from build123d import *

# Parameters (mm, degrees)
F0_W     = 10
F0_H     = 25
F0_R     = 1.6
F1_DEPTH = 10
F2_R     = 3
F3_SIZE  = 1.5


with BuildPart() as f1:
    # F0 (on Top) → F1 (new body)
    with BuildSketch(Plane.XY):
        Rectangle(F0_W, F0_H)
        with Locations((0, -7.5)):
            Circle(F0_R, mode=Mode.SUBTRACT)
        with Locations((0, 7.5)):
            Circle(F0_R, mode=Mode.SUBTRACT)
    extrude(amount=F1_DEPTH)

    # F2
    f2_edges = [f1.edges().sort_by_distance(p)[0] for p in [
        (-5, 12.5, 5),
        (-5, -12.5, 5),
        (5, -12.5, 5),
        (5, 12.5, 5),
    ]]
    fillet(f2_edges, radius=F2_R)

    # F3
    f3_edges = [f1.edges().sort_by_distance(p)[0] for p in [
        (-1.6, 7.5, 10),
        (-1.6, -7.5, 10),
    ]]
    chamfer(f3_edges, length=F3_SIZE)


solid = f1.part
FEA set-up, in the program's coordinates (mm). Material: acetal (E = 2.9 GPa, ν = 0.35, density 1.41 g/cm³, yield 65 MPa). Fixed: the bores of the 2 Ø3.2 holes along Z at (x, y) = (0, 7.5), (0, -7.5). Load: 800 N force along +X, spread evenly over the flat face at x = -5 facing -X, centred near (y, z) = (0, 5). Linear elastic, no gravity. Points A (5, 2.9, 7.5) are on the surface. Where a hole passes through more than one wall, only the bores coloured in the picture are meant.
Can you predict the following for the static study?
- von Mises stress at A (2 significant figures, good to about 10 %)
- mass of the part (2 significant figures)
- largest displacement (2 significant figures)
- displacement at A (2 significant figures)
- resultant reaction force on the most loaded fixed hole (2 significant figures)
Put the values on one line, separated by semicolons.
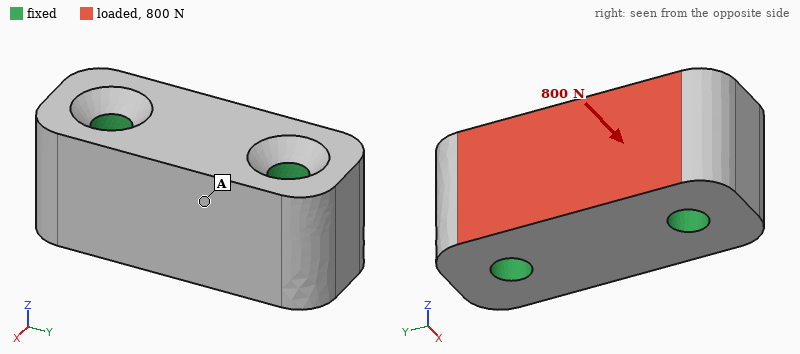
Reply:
3.1 MPa; 3.1 g; 24 µm; 12 µm; 410 N
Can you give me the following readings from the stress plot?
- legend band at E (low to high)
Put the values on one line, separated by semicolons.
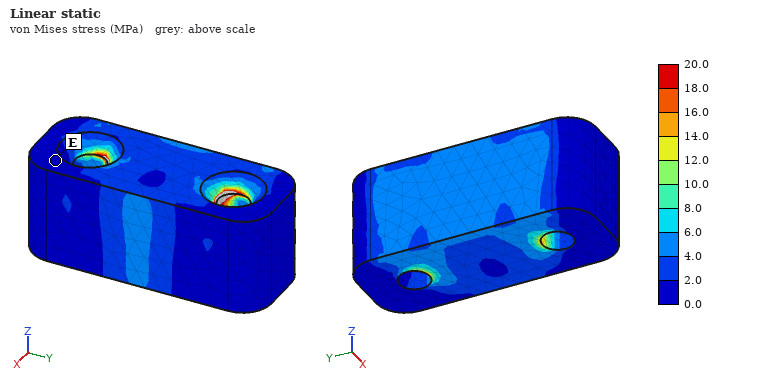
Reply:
0.0 to 2.0 MPa
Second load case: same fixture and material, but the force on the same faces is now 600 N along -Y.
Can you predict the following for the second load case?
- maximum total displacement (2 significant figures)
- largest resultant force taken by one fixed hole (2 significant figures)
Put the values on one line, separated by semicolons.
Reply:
16 µm; 340 N
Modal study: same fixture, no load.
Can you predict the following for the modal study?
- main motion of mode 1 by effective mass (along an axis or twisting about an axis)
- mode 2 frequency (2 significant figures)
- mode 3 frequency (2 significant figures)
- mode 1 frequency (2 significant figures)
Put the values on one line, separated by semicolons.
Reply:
along X; 25 kHz; 25 kHz; 23 kHz
